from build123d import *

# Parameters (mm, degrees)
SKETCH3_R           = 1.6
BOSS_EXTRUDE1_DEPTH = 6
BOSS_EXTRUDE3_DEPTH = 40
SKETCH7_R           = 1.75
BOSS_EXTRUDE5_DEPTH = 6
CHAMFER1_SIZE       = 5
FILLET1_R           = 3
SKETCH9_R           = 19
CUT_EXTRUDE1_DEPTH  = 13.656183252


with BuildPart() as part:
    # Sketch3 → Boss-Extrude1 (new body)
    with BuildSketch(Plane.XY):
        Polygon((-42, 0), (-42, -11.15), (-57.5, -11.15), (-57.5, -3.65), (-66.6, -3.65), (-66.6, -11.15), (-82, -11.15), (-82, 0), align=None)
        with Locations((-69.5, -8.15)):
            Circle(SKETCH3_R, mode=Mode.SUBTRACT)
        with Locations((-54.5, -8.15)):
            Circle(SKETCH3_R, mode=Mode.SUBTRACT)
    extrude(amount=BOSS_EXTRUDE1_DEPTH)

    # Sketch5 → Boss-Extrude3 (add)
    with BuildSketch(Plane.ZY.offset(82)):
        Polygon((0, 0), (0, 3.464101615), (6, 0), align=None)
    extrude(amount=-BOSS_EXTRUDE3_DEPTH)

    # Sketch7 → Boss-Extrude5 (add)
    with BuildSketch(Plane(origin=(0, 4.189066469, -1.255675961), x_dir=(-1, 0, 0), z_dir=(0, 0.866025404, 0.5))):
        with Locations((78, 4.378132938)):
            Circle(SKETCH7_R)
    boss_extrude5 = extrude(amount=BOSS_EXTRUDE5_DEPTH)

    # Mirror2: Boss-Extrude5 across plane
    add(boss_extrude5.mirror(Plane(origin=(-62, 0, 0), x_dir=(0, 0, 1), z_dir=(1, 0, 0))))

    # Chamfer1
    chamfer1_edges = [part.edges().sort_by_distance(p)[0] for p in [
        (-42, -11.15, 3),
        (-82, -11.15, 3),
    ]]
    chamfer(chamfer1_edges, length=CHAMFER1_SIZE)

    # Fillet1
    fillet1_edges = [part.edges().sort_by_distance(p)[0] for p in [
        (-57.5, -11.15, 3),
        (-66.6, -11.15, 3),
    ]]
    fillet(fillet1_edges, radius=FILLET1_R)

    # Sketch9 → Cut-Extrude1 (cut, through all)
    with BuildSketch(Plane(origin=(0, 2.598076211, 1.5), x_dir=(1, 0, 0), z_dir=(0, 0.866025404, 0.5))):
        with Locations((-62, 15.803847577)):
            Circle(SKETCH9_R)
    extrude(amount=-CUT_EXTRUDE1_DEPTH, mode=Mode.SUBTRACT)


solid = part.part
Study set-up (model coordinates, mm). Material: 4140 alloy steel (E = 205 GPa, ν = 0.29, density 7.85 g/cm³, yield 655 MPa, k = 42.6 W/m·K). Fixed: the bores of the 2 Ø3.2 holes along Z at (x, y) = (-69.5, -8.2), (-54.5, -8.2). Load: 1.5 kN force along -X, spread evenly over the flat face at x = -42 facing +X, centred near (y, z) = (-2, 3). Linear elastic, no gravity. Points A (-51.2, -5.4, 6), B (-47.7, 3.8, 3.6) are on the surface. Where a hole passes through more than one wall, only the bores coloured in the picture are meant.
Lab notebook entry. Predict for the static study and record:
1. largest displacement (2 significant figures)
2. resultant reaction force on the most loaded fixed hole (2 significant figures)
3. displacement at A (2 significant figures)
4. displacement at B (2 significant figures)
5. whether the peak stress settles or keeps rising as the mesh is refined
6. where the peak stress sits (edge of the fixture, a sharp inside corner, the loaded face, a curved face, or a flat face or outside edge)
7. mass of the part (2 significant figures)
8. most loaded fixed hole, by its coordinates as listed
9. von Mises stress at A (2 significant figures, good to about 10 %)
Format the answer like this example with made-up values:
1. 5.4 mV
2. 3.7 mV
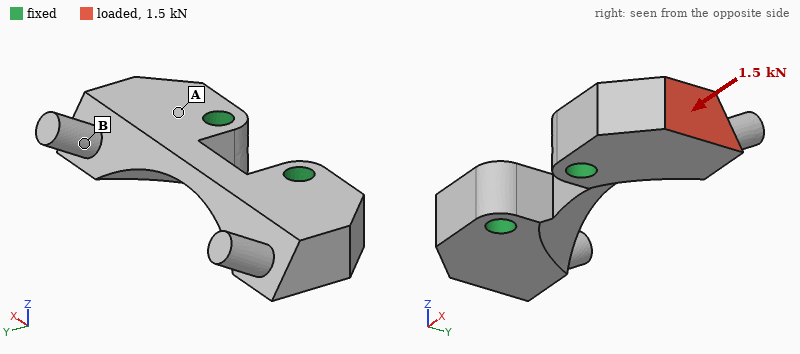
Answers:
1. 12 µm
2. 1.1 kN
3. 2.0 µm
4. 9.0 µm
5. keeps rising
6. edge of the fixture
7. 18 g
8. (-54.5, -8.2)
9. 34 MPa
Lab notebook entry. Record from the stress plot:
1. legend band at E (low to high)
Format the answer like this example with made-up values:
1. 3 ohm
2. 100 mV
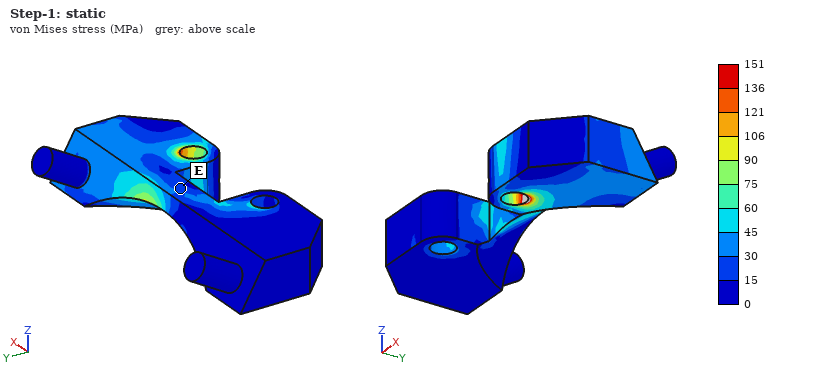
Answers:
1. 15 to 30 MPa
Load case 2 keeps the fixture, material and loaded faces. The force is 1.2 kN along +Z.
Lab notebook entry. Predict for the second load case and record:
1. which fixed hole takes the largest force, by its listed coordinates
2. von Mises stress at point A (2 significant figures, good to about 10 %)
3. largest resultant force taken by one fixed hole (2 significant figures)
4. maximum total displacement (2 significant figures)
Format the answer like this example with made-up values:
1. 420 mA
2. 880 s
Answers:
1. (-54.5, -8.2)
2. 200 MPa
3. 1.3 kN
4. 41 µm
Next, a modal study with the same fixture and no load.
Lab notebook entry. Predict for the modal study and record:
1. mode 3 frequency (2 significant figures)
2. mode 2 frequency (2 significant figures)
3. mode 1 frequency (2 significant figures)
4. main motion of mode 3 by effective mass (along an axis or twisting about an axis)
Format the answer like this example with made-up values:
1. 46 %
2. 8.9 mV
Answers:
1. 22 kHz
2. 20 kHz
3. 20 kHz
4. along X
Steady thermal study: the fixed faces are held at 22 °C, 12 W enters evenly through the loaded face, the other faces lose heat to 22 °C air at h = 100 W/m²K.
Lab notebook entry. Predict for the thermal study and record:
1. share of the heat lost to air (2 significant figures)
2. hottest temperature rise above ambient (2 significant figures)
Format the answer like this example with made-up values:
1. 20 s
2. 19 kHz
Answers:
1. 13 %
2. 60 K
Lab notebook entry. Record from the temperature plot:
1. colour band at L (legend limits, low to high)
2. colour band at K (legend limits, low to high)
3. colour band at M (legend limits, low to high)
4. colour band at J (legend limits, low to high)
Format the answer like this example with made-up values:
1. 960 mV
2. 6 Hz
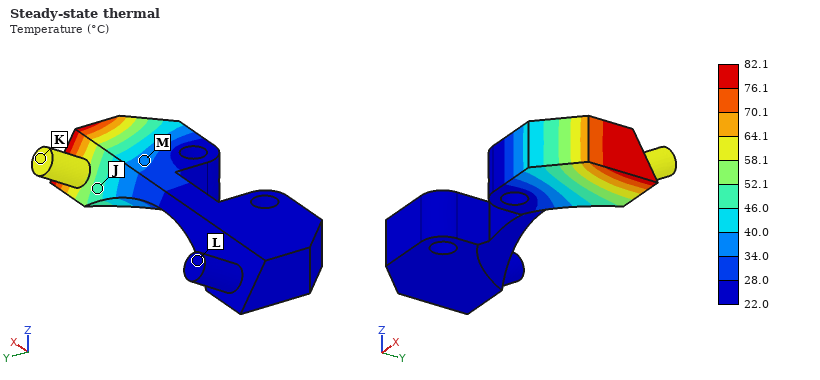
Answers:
1. 22.0 to 28.0 °C
2. 58.1 to 64.1 °C
3. 34.0 to 40.0 °C
4. 46.0 to 52.1 °C
